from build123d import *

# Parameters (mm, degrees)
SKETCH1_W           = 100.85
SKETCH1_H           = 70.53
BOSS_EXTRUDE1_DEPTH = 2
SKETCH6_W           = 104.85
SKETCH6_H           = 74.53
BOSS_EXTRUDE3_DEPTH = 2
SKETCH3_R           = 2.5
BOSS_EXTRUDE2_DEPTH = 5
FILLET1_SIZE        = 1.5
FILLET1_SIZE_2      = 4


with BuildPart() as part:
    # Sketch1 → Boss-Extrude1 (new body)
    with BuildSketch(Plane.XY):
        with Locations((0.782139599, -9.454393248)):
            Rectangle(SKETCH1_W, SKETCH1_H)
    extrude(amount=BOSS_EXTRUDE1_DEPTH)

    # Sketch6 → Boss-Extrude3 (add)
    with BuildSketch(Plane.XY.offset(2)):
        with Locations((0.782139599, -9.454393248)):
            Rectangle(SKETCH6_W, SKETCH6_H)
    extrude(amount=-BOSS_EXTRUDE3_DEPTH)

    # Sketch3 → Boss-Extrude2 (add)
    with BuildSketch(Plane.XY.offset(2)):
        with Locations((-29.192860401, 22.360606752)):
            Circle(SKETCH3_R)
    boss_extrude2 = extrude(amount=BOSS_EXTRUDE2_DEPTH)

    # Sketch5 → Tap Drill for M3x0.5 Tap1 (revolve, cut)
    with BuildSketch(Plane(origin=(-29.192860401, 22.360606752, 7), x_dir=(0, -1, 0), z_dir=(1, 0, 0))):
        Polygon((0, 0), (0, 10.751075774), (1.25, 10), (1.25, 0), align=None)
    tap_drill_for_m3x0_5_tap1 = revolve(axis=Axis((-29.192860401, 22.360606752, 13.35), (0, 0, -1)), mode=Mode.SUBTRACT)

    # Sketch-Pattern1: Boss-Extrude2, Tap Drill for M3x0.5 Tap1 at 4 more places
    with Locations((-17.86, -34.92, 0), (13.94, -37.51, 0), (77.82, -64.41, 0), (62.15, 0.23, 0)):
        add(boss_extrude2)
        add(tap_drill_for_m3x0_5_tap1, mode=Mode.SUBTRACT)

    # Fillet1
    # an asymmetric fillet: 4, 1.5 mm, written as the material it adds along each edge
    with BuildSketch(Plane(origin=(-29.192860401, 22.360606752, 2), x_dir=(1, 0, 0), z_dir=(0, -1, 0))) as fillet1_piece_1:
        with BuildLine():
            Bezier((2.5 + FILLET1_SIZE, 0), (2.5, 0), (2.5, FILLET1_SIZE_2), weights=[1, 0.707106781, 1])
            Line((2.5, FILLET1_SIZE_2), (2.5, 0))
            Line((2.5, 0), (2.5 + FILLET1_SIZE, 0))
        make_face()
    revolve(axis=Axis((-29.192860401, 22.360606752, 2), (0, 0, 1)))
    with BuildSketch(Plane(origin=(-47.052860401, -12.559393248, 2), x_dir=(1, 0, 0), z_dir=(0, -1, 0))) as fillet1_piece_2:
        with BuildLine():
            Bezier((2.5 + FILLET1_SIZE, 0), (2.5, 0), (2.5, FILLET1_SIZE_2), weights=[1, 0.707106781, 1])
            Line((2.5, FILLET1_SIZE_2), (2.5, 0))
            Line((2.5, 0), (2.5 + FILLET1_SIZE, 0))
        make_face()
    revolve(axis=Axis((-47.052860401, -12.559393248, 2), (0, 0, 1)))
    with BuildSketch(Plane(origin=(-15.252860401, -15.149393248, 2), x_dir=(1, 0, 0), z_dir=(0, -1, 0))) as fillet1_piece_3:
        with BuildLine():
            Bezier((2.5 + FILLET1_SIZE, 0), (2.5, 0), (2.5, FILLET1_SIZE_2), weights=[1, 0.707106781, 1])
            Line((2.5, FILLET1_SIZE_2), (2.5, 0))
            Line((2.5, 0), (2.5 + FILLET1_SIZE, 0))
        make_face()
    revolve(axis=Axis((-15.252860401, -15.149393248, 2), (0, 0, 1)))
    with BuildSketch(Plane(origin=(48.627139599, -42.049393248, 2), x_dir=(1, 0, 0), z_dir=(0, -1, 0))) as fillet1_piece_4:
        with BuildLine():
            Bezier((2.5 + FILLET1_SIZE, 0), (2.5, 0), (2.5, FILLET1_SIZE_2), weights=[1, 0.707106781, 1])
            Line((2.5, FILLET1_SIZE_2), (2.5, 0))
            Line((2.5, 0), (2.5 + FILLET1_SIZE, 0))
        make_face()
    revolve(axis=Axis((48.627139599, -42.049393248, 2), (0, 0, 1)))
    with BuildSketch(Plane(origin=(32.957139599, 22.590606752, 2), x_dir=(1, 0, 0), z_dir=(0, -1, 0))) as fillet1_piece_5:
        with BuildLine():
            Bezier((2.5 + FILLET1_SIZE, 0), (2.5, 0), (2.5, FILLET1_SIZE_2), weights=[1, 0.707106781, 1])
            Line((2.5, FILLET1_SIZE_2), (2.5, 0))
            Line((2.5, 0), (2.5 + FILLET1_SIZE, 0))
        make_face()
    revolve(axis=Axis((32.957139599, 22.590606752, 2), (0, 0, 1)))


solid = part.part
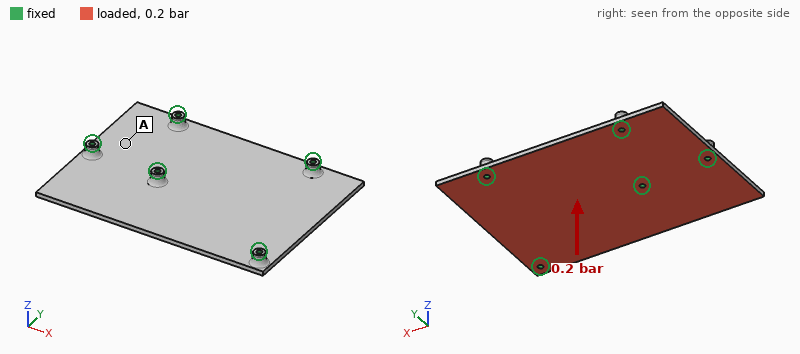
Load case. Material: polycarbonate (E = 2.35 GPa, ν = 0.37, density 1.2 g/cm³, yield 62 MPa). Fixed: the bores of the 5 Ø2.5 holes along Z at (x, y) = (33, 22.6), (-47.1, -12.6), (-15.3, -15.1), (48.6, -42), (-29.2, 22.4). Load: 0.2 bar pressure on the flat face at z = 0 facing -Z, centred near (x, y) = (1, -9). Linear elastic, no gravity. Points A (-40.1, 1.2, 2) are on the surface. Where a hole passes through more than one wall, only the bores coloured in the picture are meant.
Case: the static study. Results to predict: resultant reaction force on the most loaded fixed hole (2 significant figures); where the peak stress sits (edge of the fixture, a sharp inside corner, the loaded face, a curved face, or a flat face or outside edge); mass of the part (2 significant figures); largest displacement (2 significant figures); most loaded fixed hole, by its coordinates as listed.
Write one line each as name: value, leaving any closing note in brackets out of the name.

resultant reaction force on the most loaded fixed hole: 57 N
where the peak stress sits: a curved face
mass of the part: 19 g
largest displacement: 1.5 mm
most loaded fixed hole, by its coordinates as listed: (-15.3, -15.1)
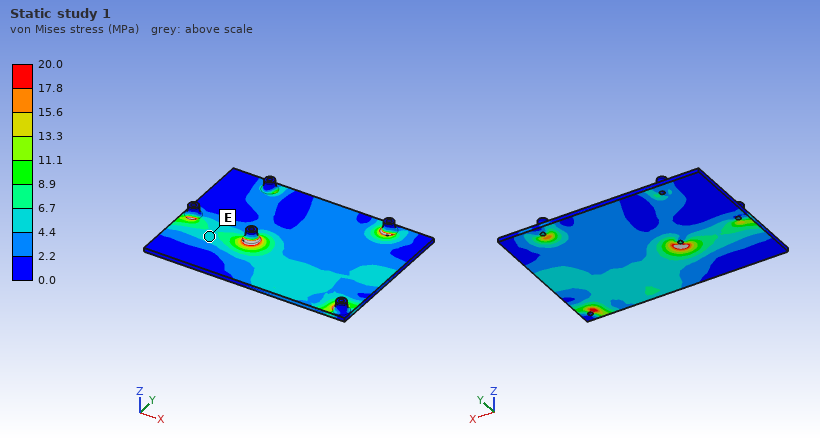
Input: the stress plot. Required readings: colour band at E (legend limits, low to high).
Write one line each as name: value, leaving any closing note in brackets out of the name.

colour band at E: 4.4 to 6.7 MPa
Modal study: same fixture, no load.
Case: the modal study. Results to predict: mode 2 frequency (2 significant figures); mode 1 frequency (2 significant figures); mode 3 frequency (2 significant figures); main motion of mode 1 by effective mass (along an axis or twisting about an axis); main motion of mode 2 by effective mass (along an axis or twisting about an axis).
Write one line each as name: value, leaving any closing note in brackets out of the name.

mode 2 frequency: 590 Hz
mode 1 frequency: 460 Hz
mode 3 frequency: 690 Hz
main motion of mode 1 by effective mass: along Z
main motion of mode 2 by effective mass: along Z
